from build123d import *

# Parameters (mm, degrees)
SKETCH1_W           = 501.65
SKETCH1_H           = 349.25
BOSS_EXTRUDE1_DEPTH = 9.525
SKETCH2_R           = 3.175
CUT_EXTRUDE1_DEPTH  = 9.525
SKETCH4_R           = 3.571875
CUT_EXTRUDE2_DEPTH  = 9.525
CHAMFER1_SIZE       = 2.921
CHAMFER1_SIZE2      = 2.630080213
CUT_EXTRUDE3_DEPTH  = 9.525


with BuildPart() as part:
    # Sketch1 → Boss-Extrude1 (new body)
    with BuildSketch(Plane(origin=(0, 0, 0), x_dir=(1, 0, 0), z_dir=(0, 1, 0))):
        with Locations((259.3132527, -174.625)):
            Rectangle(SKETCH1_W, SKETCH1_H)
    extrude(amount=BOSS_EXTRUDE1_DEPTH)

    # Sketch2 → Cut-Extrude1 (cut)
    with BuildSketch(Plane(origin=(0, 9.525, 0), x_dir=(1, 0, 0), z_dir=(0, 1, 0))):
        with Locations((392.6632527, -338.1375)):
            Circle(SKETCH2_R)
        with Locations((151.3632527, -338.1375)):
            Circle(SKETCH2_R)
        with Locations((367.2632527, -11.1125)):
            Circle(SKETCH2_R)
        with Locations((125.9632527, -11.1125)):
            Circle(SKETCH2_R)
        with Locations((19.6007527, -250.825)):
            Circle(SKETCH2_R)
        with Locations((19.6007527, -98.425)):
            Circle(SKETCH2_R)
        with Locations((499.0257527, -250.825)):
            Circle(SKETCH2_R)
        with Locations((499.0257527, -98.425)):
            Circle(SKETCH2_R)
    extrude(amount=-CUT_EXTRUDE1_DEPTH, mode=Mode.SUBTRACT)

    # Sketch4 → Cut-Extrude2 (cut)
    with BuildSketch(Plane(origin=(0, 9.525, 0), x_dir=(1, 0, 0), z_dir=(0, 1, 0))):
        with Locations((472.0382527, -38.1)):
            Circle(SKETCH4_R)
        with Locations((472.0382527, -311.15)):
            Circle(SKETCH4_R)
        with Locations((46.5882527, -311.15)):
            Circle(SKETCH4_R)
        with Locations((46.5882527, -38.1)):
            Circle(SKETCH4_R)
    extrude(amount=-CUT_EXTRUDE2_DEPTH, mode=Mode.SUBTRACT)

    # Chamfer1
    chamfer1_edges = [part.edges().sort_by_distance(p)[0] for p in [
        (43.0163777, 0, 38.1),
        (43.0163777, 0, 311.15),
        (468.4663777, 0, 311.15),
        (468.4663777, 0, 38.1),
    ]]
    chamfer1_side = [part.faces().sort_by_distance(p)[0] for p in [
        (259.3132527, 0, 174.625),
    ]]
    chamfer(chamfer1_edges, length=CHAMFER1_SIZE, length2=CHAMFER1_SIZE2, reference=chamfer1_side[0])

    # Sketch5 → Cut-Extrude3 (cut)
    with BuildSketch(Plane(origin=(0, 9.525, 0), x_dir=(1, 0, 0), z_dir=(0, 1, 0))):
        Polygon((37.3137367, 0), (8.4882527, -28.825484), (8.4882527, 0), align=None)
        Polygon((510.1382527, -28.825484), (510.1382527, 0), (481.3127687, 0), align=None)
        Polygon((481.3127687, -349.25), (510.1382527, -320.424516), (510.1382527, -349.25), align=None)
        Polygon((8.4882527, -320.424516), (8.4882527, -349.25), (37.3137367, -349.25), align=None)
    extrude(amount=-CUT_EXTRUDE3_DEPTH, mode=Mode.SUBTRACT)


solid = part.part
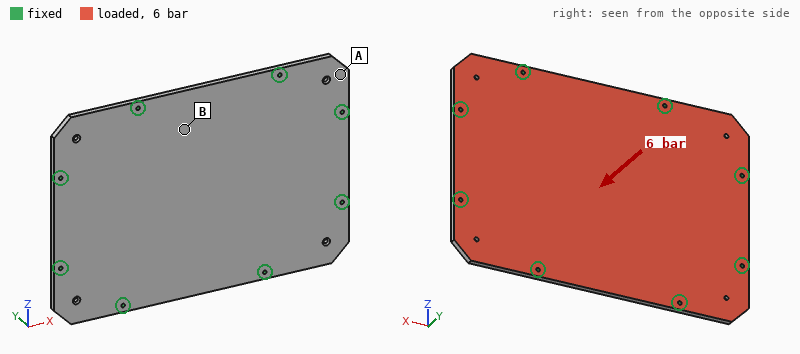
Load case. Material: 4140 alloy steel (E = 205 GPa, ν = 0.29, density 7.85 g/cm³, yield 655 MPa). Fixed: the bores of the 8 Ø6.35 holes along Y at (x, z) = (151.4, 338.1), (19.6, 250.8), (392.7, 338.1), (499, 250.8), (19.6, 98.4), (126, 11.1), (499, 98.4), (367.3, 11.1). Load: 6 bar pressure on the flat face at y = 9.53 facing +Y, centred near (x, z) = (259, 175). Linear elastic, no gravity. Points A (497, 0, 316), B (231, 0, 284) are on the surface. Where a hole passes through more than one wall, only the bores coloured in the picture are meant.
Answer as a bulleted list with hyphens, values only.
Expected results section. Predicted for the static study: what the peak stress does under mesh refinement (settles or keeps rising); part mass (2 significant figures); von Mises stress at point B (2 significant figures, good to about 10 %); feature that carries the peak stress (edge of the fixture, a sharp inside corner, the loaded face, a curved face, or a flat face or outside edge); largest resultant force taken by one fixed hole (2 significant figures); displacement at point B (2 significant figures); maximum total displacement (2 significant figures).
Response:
- keeps rising
- 13 kg
- 120 MPa
- edge of the fixture
- 18 kN
- 1.3 mm
- 2.2 mm
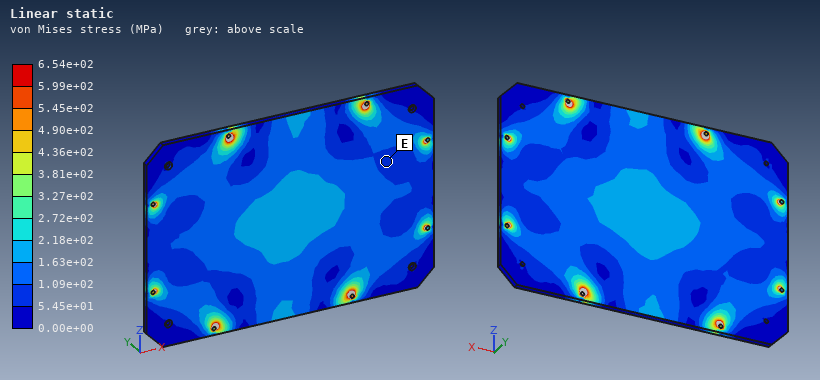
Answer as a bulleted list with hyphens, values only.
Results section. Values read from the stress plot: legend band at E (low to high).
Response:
- 5.45e+01 to 1.09e+02 MPa
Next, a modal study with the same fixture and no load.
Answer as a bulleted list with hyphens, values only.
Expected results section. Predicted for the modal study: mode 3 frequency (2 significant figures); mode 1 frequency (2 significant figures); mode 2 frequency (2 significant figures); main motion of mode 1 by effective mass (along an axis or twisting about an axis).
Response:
- 780 Hz
- 380 Hz
- 720 Hz
- along Y
